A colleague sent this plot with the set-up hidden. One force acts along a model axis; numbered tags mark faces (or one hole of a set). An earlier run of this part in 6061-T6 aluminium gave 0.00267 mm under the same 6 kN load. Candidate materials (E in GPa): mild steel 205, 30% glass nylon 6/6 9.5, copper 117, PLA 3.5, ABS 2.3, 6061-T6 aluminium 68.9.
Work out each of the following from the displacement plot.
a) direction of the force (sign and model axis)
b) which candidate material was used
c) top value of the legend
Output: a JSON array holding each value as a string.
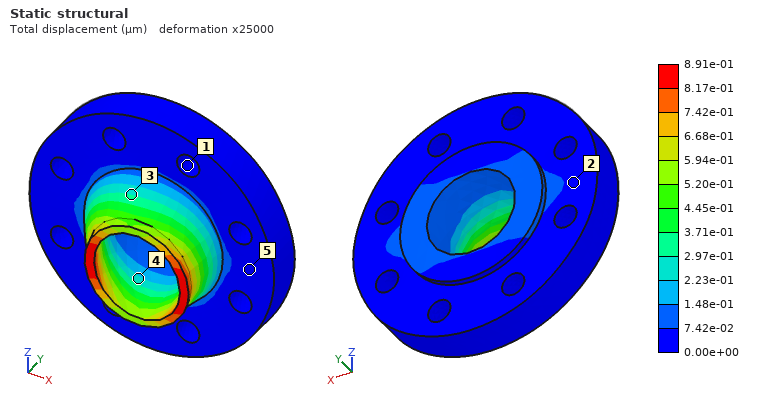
["+X", "mild steel", "8.91e-01 µm"]
